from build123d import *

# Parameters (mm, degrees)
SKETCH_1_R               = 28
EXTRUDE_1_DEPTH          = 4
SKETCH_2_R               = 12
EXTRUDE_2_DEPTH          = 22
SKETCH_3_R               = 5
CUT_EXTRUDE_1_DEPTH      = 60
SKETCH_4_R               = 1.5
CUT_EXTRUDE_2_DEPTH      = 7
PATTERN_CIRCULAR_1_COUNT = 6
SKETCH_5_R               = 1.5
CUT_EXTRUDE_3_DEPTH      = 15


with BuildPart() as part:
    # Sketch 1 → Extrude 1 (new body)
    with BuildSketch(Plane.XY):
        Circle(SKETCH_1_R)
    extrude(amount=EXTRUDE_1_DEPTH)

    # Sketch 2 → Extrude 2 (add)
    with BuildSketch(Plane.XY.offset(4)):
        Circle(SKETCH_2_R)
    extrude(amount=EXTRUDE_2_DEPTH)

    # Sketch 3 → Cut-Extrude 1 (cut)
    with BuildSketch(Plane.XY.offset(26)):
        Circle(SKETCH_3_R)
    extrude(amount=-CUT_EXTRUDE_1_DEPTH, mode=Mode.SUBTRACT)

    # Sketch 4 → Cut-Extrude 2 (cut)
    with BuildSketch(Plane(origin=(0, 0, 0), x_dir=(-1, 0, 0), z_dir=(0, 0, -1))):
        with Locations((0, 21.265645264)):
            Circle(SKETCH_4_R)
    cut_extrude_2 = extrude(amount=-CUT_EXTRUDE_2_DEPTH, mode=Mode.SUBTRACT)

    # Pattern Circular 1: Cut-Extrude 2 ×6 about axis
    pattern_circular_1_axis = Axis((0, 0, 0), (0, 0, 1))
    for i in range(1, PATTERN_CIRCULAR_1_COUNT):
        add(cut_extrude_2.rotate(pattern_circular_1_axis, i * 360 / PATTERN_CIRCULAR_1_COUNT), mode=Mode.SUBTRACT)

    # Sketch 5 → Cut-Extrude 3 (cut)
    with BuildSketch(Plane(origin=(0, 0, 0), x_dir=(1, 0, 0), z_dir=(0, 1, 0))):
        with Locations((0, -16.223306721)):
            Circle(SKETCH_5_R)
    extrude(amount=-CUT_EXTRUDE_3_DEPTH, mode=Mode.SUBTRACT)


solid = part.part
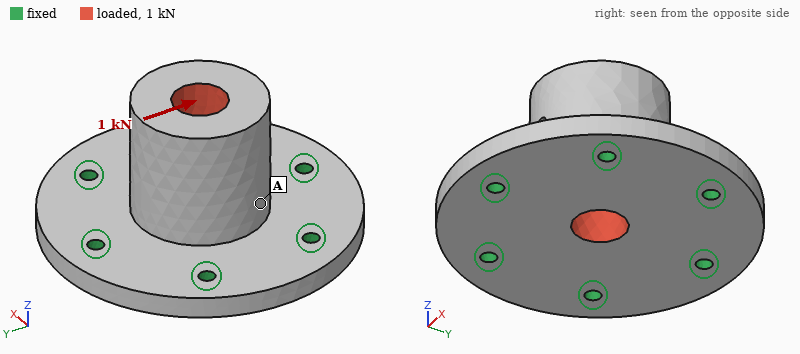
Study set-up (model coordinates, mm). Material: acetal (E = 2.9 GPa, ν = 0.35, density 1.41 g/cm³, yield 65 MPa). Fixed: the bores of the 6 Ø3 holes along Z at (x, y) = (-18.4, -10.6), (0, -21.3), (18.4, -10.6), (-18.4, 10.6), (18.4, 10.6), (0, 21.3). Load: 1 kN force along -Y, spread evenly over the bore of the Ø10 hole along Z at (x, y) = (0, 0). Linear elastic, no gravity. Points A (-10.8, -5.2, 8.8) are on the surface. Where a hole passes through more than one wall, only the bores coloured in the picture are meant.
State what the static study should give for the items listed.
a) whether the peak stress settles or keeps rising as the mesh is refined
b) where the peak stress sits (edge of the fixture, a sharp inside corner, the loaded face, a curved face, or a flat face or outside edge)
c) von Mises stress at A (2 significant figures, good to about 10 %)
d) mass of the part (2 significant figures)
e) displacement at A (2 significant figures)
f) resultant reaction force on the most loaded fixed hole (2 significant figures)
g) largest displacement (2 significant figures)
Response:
keeps rising
edge of the fixture
3.6 MPa
25 g
0.098 mm
330 N
0.31 mm
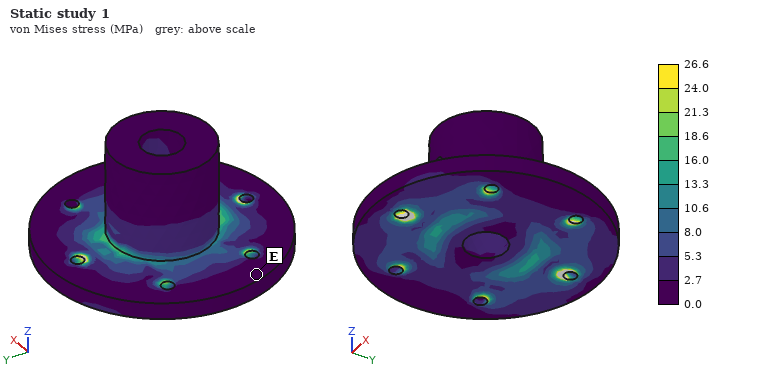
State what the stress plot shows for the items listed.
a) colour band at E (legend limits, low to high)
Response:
0.0 to 2.7 MPa
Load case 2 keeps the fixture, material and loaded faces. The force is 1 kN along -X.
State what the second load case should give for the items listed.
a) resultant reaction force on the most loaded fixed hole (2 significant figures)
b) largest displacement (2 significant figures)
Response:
290 N
0.31 mm
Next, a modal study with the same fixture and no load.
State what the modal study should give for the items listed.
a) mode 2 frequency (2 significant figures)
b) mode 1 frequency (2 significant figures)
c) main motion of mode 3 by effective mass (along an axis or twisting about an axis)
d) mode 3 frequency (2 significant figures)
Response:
2800 Hz
2800 Hz
along Z
3600 Hz
